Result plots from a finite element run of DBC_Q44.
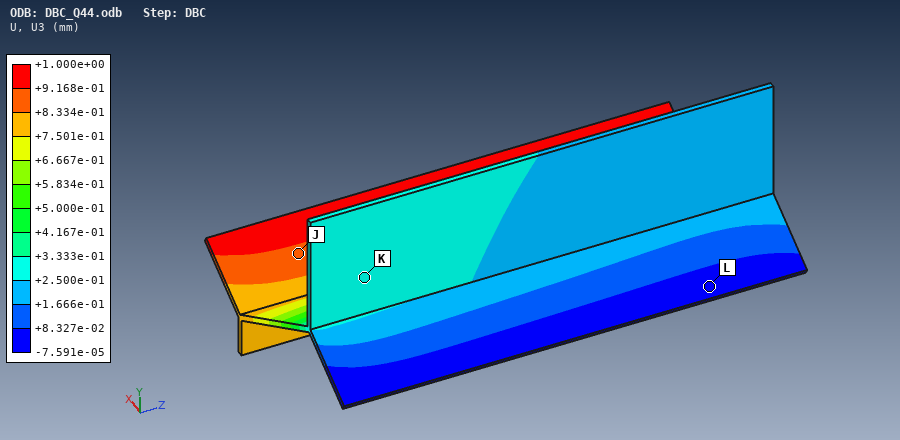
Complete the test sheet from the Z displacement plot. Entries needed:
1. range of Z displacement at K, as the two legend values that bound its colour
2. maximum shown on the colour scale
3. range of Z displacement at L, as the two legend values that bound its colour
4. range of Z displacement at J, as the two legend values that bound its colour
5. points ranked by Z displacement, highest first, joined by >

+2.500e-01 to +3.333e-01 mm
+1.000e+00 mm
-7.591e-05 to +8.327e-02 mm
+8.334e-01 to +9.168e-01 mm
J > K > L
